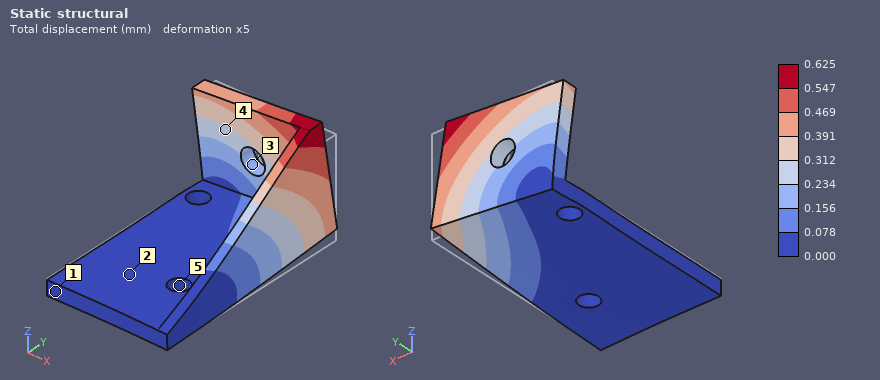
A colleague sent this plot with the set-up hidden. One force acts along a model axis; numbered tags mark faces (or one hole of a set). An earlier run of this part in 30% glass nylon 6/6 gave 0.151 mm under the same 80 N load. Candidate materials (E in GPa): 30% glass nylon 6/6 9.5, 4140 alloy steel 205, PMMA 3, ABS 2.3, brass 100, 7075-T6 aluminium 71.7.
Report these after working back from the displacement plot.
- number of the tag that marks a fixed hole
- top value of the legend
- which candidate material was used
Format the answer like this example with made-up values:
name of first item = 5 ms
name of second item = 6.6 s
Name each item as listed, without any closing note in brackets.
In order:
number of the tag that marks a fixed hole = 5
top value of the legend = 0.625 mm
which candidate material was used = ABS
